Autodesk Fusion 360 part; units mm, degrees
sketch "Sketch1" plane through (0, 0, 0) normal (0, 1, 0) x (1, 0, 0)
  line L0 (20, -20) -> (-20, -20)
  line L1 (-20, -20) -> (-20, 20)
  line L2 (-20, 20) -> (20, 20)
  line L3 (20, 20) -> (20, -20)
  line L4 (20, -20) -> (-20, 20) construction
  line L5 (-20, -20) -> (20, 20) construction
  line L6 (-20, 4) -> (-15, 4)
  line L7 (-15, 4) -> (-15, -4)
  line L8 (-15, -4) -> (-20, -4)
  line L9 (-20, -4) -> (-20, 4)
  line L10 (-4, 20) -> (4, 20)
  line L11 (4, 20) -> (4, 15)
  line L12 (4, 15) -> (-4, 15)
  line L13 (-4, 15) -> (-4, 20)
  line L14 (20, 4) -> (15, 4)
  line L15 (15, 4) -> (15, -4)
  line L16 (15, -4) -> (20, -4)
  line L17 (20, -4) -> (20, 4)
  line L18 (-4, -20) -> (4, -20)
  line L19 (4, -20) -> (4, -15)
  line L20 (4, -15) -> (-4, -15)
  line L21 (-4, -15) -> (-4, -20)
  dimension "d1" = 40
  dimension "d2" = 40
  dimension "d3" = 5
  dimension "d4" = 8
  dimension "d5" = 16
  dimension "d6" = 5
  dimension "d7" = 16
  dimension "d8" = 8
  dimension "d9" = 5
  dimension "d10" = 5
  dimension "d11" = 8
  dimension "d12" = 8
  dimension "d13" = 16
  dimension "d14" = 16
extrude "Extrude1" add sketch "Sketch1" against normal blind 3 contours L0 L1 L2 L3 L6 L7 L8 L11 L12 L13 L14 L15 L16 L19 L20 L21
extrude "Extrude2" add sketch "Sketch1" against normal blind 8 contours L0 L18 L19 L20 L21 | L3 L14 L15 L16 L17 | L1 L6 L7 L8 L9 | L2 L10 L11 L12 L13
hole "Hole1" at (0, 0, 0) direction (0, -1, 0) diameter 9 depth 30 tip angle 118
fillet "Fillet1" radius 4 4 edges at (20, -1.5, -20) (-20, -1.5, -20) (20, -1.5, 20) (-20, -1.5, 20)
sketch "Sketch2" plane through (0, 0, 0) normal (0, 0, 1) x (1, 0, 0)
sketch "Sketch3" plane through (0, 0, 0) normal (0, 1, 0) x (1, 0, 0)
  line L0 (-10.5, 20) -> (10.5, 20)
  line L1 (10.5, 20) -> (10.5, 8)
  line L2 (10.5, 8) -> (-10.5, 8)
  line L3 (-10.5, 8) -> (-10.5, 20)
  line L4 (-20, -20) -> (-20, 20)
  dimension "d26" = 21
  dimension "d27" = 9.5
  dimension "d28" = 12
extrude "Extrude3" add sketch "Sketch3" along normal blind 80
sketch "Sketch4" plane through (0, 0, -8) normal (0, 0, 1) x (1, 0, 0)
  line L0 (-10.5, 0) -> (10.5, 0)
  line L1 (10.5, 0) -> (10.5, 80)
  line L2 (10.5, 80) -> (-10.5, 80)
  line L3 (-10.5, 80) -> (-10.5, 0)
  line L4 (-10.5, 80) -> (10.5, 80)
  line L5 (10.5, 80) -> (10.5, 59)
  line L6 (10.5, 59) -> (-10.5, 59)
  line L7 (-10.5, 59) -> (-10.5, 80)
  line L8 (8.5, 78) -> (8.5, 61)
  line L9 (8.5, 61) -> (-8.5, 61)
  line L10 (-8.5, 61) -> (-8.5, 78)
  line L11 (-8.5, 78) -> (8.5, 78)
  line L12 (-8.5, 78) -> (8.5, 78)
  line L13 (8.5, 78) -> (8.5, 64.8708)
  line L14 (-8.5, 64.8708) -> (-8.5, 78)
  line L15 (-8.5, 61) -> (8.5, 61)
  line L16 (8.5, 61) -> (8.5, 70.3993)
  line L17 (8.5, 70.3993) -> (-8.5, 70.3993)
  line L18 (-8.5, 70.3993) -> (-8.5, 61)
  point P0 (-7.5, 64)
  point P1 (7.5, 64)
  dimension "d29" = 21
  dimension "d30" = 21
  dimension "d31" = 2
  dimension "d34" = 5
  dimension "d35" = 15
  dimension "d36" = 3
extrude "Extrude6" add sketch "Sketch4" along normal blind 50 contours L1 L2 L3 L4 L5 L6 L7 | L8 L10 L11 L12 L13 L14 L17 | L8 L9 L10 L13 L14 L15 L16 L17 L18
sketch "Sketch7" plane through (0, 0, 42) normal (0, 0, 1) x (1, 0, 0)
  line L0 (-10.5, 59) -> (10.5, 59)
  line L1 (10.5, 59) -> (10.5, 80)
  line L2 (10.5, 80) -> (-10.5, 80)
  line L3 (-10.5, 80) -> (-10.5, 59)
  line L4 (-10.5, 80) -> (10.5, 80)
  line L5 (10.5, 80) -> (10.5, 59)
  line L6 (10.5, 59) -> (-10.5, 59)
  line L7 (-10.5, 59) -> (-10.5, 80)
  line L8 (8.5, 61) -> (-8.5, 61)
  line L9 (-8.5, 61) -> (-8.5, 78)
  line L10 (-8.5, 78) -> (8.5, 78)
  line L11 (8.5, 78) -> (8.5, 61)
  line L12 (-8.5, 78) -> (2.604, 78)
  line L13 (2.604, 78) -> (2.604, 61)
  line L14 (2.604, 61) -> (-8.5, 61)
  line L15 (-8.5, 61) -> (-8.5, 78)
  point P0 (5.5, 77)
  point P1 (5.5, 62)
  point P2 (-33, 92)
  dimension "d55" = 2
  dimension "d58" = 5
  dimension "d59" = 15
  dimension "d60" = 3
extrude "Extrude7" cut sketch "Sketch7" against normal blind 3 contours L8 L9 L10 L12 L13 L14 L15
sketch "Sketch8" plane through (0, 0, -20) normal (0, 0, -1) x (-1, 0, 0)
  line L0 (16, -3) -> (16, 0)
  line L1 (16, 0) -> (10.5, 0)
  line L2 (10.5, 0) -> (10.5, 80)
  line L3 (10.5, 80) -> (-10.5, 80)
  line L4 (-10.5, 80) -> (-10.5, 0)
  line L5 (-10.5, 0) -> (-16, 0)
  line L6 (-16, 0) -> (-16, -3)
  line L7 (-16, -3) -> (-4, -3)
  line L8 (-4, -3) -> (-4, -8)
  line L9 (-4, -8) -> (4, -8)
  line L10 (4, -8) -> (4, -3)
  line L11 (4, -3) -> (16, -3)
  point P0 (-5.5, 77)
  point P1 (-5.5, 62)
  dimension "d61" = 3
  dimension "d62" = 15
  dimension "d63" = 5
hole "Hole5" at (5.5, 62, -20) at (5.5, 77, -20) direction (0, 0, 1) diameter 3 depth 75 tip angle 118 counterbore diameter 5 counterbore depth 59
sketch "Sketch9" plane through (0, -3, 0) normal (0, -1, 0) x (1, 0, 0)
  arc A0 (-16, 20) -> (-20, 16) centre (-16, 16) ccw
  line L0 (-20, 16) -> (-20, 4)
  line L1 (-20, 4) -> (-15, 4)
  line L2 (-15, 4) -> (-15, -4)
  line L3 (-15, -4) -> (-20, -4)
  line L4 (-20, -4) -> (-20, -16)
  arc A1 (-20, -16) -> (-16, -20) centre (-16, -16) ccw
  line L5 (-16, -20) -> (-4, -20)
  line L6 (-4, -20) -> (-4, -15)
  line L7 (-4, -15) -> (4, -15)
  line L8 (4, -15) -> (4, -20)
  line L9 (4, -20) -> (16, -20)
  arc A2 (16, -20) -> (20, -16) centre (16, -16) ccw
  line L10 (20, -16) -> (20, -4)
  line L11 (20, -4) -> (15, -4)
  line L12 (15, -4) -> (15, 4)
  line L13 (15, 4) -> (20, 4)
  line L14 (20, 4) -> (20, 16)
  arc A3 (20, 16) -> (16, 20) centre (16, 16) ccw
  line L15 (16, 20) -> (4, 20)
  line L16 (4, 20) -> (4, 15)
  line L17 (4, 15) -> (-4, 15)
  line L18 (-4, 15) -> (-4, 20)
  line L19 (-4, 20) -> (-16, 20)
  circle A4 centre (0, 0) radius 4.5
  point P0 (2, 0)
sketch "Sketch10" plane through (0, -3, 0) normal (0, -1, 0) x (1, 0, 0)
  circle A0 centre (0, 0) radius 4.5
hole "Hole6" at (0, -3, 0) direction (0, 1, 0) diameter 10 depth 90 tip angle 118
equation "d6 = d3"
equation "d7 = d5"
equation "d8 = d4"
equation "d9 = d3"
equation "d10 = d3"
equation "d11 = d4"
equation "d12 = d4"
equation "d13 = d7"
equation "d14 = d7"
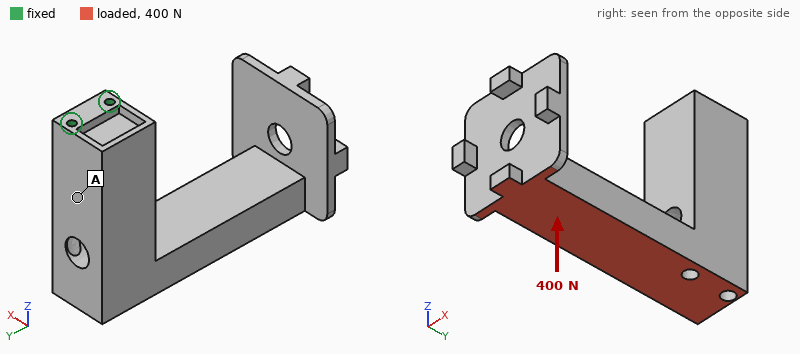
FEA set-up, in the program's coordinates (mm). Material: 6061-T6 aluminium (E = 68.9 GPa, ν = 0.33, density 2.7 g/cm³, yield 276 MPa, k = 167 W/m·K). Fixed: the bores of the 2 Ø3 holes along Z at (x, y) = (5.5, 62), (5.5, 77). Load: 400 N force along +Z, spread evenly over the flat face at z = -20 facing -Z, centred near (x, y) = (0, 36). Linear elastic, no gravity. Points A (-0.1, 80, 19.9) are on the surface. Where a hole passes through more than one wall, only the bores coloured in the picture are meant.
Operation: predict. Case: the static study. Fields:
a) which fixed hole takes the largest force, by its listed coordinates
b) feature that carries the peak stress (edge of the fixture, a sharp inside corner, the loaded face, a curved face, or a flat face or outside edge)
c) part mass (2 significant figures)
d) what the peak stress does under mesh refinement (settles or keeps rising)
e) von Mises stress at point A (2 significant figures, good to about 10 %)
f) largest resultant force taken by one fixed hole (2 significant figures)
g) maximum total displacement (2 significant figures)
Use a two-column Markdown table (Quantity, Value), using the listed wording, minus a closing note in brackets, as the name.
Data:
| Quantity | Value |
|---|---|
| which fixed hole takes the largest force, by its listed coordinates | (5.5, 62) |
| feature that carries the peak stress | edge of the fixture |
| part mass | 120 g |
| what the peak stress does under mesh refinement | keeps rising |
| von Mises stress at point A | 8.4 MPa |
| largest resultant force taken by one fixed hole | 1.0 kN |
| maximum total displacement | 0.22 mm |
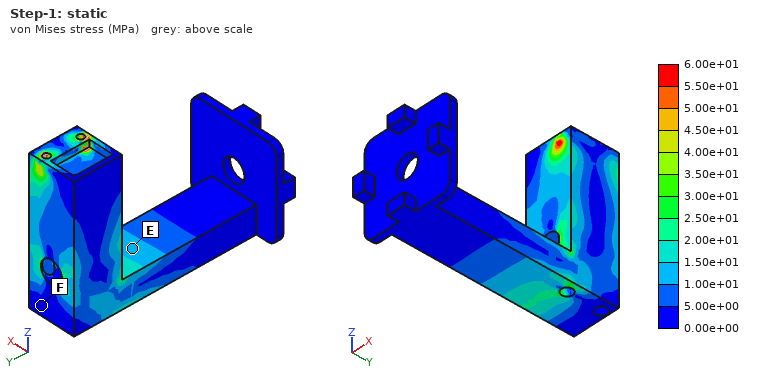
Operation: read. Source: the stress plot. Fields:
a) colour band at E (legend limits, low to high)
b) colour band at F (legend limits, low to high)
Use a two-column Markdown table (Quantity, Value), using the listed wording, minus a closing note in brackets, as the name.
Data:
| Quantity | Value |
|---|---|
| colour band at E | 1.00e+01 to 1.50e+01 MPa |
| colour band at F | 0.00e+00 to 5.00e+00 MPa |
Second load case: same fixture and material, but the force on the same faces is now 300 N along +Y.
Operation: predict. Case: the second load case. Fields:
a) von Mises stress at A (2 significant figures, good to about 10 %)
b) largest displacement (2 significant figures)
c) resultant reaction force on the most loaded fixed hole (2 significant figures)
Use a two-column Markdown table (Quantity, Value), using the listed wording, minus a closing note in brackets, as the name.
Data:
| Quantity | Value |
|---|---|
| von Mises stress at A | 8.8 MPa |
| largest displacement | 0.13 mm |
| resultant reaction force on the most loaded fixed hole | 1.2 kN |
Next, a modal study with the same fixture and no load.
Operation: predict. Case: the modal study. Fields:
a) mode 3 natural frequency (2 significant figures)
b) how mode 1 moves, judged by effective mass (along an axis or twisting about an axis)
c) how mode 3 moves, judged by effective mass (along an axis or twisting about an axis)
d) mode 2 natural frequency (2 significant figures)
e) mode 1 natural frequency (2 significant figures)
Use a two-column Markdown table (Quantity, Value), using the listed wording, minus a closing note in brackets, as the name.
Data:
| Quantity | Value |
|---|---|
| mode 3 natural frequency | 1400 Hz |
| how mode 1 moves, judged by effective mass | along X |
| how mode 3 moves, judged by effective mass | twisting about Z |
| mode 2 natural frequency | 860 Hz |
| mode 1 natural frequency | 510 Hz |
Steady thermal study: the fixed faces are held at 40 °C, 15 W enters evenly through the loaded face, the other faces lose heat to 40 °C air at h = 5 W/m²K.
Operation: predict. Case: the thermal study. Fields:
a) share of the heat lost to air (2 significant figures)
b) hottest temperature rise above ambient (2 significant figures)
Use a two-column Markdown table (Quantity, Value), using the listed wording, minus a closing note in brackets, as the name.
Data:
| Quantity | Value |
|---|---|
| share of the heat lost to air | 8.1 % |
| hottest temperature rise above ambient | 28 K |
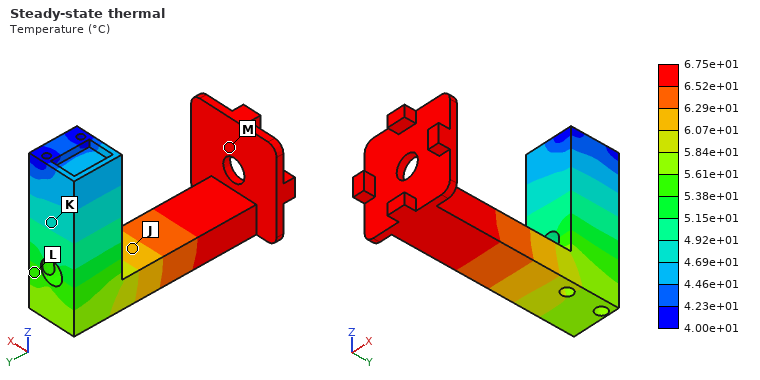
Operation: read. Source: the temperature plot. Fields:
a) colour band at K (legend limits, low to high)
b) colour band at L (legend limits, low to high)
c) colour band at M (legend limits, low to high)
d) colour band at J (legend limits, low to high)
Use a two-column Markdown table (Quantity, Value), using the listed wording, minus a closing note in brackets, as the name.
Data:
| Quantity | Value |
|---|---|
| colour band at K | 4.69e+01 to 4.92e+01 °C |
| colour band at L | 5.38e+01 to 5.61e+01 °C |
| colour band at M | 6.52e+01 to 6.75e+01 °C |
| colour band at J | 6.07e+01 to 6.29e+01 °C |
